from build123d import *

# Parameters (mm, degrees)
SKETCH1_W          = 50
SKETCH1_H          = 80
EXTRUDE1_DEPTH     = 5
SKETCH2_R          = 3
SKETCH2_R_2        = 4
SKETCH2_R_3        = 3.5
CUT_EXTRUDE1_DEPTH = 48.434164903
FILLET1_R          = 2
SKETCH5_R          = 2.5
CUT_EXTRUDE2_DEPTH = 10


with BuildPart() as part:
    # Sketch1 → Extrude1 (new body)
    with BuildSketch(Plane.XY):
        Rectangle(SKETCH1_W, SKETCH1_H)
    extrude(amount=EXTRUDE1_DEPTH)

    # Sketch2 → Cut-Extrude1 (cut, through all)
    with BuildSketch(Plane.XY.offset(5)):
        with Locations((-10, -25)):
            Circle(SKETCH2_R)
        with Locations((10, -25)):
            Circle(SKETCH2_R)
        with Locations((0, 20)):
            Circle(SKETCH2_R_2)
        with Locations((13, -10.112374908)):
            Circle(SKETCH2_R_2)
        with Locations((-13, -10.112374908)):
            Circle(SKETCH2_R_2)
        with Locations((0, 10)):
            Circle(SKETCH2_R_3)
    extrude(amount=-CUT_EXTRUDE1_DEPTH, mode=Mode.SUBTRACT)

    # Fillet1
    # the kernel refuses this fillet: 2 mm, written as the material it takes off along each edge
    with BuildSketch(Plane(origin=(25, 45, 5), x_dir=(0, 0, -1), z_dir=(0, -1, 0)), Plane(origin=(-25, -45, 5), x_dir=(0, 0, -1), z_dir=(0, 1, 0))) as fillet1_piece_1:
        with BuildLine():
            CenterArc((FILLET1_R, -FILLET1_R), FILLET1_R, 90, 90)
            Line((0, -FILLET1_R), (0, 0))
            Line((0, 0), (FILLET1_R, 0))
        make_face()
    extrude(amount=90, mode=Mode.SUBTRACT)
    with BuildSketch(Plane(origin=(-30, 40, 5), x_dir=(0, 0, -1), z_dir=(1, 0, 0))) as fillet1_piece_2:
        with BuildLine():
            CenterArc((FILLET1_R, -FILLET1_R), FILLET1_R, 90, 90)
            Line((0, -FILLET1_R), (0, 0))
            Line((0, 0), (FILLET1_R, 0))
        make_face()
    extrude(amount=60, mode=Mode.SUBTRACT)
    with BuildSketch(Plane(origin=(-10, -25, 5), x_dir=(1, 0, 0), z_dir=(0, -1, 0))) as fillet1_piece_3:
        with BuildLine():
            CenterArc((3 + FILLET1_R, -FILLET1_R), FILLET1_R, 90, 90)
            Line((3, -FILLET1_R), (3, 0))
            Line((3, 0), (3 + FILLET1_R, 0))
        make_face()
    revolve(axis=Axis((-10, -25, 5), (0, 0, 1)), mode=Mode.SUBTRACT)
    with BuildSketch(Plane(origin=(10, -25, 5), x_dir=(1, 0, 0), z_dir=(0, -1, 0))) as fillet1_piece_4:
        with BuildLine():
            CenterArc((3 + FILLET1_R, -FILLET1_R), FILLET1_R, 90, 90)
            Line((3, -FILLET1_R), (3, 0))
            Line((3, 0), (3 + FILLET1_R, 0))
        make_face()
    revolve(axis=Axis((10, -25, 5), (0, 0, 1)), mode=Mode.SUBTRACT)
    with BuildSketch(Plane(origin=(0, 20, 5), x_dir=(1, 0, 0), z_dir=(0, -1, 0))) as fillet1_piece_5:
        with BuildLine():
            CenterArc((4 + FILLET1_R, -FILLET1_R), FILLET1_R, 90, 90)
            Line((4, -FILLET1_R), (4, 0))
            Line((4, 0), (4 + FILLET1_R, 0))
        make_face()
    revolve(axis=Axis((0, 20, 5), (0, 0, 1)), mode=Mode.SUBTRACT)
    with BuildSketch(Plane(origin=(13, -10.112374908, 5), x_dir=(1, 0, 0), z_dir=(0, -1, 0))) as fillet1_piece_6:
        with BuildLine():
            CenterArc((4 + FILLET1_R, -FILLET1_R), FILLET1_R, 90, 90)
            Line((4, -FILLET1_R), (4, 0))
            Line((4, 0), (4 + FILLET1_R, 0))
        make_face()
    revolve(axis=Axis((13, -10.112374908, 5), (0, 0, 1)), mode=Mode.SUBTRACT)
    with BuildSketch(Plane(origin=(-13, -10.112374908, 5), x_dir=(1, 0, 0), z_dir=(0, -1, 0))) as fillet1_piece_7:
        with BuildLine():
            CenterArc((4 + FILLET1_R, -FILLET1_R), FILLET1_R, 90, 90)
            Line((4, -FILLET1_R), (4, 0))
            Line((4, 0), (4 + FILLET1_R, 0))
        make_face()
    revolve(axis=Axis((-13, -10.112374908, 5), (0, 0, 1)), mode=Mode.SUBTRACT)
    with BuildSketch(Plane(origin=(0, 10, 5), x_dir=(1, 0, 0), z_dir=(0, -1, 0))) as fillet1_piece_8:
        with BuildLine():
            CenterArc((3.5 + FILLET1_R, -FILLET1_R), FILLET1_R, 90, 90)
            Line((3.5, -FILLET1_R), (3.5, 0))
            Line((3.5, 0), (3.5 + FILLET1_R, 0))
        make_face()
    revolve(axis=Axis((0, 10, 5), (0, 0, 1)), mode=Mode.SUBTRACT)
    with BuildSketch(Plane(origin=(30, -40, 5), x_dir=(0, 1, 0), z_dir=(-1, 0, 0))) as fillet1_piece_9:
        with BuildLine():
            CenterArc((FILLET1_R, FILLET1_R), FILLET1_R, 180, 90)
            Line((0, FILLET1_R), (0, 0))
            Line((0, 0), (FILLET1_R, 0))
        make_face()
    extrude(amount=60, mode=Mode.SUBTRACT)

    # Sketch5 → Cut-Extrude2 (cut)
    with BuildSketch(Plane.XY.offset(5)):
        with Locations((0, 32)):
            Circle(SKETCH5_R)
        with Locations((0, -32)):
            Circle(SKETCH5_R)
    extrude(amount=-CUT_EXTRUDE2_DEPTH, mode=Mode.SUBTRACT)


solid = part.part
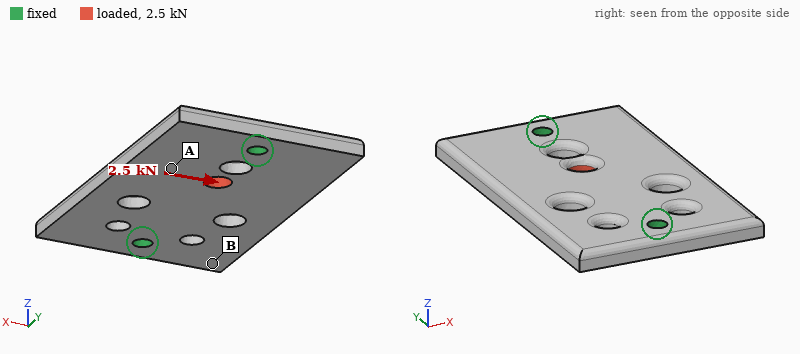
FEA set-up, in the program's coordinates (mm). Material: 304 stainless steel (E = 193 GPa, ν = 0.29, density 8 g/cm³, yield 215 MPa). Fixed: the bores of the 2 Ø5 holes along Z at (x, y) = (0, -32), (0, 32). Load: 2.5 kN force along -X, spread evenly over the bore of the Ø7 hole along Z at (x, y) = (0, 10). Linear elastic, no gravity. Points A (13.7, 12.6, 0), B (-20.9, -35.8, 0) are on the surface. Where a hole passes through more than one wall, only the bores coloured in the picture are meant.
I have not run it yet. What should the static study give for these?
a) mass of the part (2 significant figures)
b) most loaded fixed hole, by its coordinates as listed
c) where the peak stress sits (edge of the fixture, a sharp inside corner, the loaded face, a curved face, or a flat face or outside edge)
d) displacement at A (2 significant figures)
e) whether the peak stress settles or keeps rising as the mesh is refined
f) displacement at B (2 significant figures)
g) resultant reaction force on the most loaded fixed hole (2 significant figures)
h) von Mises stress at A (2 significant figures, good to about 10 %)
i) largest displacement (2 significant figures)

150 g
(0, 32)
edge of the fixture
5.4 µm
keeps rising
1.8 µm
1.6 kN
15 MPa
7.4 µm
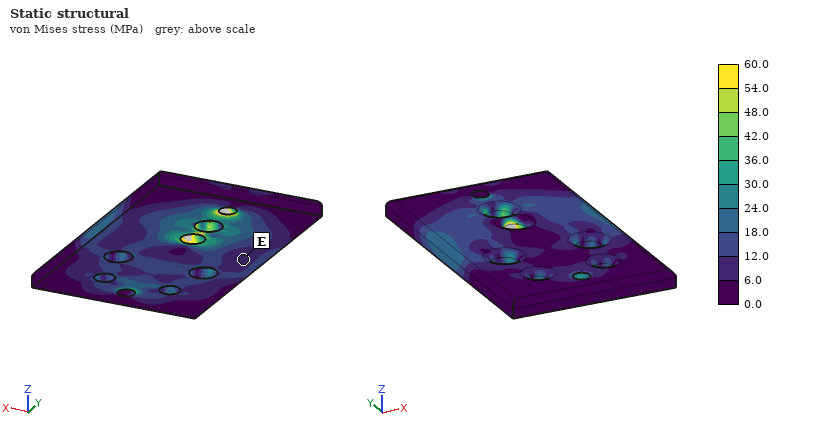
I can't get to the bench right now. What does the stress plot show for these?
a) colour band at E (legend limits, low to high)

6.0 to 12.0 MPa
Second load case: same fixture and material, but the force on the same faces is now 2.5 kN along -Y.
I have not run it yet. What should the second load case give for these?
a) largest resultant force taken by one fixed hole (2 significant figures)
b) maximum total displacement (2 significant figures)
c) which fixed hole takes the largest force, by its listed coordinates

1.4 kN
4.6 µm
(0, 32)
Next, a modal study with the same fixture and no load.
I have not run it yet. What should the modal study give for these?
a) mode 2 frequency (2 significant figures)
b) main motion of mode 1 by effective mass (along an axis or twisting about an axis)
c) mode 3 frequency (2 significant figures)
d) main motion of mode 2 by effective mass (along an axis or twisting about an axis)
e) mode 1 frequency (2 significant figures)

4200 Hz
twisting about Y
6900 Hz
along Z
3600 Hz
